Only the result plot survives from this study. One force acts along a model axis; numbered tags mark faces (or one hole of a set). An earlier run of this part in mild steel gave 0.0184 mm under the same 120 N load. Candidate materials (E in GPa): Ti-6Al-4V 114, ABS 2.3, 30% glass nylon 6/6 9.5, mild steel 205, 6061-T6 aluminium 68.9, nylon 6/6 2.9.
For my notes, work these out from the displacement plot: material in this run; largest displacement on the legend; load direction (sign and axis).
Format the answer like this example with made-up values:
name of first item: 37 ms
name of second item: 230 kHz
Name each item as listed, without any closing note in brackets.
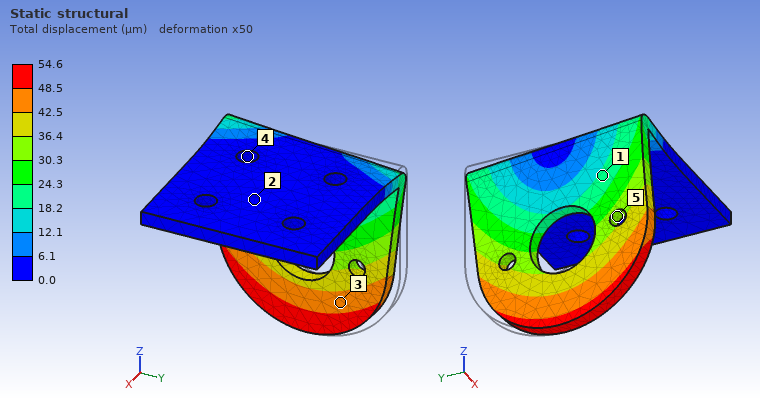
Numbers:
material in this run: 6061-T6 aluminium
largest displacement on the legend: 54.6 µm
load direction: -Y
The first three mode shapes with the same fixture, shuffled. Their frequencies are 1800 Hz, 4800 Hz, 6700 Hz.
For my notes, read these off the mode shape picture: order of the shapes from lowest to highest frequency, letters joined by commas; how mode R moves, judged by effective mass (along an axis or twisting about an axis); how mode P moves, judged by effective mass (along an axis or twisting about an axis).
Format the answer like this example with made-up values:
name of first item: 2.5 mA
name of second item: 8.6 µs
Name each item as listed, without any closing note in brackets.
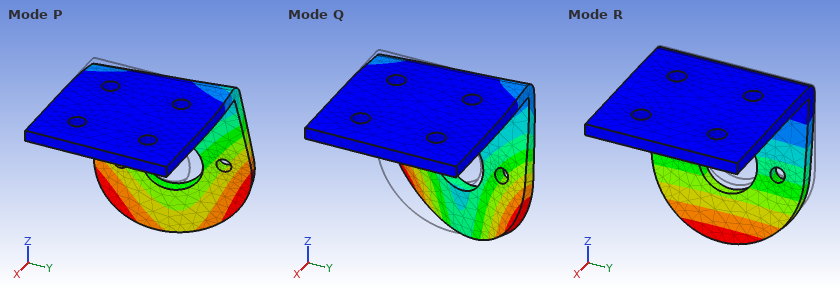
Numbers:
order of the shapes from lowest to highest frequency, letters joined by commas: R, P, Q
how mode R moves, judged by effective mass: along X
how mode P moves, judged by effective mass: along Y
